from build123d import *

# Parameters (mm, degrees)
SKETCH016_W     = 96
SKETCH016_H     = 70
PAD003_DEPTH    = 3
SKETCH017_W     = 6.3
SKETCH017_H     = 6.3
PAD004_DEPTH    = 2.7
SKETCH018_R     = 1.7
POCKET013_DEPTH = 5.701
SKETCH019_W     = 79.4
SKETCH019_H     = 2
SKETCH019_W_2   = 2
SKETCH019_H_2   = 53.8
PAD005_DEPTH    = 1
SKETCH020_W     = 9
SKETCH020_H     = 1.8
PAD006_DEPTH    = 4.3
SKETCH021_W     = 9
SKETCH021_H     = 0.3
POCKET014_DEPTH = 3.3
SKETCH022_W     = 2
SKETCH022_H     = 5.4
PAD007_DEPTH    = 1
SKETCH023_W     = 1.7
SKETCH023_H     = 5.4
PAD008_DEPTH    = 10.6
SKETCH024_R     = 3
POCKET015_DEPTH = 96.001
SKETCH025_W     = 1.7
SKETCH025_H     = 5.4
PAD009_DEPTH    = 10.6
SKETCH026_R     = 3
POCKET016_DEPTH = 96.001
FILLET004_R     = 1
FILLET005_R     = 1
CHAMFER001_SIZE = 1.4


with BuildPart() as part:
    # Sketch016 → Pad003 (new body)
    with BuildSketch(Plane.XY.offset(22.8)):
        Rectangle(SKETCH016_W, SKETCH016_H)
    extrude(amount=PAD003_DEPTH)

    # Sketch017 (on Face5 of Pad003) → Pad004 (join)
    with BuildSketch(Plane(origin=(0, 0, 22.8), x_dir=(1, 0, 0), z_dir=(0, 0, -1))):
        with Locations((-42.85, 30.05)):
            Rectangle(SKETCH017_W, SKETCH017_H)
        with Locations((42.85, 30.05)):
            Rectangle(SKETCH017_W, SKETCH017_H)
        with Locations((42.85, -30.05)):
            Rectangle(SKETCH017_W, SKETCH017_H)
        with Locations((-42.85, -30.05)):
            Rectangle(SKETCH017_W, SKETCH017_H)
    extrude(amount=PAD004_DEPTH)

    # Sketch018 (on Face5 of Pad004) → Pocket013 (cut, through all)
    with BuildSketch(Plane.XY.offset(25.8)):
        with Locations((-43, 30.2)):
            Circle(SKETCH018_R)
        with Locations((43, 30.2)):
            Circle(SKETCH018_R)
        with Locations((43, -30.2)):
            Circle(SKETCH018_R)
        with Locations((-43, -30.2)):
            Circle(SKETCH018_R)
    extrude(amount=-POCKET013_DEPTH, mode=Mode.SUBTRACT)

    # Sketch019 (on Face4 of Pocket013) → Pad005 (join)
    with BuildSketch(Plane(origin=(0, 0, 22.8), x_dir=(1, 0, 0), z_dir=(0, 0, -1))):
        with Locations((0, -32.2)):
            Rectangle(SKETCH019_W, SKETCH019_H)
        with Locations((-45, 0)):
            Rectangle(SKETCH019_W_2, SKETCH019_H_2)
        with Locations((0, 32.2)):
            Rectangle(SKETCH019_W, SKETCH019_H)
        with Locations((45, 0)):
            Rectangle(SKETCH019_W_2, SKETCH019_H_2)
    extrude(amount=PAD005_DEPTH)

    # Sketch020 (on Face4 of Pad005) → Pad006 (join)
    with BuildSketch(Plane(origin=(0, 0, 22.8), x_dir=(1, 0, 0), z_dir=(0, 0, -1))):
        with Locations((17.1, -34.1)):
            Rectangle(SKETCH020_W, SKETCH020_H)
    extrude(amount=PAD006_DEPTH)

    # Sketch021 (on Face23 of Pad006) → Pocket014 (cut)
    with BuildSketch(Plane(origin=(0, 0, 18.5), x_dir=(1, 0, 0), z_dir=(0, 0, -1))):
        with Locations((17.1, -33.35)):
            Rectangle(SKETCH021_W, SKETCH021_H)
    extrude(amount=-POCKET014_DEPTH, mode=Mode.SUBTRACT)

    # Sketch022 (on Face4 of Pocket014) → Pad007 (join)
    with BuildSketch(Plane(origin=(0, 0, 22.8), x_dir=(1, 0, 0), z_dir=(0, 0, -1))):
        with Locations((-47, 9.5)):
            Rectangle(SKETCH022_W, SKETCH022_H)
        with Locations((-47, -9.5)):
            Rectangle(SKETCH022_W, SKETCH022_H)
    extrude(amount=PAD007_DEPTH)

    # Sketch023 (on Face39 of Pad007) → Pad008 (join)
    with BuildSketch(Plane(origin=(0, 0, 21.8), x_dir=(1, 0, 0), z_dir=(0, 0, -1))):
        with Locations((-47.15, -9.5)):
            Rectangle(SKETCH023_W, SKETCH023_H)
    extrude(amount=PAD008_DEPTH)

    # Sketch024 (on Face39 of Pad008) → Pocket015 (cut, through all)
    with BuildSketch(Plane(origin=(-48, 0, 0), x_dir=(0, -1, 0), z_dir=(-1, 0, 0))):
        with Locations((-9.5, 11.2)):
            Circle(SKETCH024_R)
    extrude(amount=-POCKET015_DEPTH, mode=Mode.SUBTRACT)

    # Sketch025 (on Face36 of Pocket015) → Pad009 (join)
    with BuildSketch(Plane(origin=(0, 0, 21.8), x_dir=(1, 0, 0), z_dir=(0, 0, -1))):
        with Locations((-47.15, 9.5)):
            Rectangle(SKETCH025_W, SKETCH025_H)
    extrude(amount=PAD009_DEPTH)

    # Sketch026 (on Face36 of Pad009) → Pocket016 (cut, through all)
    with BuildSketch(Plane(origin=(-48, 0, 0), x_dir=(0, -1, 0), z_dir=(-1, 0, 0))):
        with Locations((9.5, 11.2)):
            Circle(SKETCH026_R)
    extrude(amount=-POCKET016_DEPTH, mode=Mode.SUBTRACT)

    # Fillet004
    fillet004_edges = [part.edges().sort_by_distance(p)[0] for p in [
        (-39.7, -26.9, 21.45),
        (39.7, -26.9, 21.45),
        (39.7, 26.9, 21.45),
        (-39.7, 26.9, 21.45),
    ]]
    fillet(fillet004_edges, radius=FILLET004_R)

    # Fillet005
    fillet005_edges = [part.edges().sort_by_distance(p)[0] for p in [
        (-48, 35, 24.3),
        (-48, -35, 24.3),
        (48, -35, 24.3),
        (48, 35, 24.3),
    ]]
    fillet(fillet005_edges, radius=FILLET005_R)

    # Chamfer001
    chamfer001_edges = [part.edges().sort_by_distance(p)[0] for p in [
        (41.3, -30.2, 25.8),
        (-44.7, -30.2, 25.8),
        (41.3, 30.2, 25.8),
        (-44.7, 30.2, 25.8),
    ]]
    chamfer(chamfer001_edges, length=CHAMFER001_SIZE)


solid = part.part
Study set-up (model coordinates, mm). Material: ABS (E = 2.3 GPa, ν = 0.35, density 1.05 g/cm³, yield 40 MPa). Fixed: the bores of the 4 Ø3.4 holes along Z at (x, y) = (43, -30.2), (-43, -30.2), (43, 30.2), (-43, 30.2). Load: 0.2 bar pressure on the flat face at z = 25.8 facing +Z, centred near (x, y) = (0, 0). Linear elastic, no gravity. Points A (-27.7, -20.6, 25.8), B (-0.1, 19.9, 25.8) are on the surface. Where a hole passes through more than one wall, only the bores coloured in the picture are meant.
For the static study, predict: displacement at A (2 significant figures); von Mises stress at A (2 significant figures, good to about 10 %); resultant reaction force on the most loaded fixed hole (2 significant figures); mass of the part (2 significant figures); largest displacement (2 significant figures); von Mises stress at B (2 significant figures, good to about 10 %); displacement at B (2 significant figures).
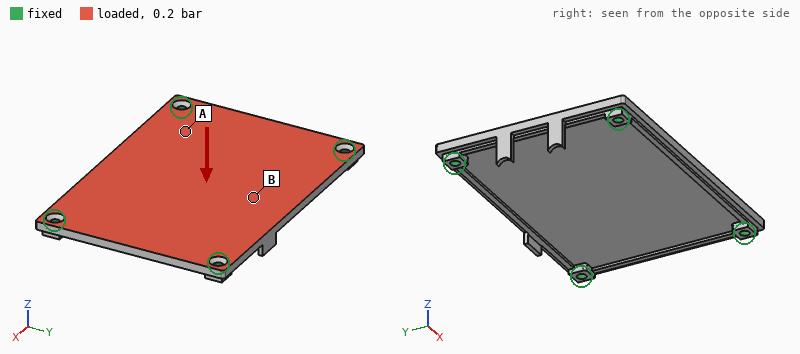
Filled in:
0.34 mm
1.2 MPa
48 N
22 g
0.80 mm
4.5 MPa
0.72 mm
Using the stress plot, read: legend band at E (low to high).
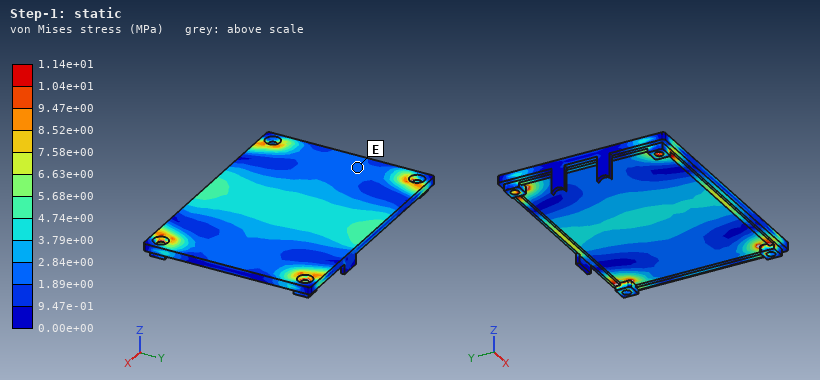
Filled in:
1.89e+00 to 2.84e+00 MPa
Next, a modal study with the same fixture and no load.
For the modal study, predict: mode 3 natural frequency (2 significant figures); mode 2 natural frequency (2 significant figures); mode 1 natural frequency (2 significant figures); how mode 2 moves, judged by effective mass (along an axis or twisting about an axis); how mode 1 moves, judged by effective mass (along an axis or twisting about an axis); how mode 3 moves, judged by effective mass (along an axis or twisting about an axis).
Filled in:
1200 Hz
830 Hz
520 Hz
twisting about X
along Z
twisting about Y
